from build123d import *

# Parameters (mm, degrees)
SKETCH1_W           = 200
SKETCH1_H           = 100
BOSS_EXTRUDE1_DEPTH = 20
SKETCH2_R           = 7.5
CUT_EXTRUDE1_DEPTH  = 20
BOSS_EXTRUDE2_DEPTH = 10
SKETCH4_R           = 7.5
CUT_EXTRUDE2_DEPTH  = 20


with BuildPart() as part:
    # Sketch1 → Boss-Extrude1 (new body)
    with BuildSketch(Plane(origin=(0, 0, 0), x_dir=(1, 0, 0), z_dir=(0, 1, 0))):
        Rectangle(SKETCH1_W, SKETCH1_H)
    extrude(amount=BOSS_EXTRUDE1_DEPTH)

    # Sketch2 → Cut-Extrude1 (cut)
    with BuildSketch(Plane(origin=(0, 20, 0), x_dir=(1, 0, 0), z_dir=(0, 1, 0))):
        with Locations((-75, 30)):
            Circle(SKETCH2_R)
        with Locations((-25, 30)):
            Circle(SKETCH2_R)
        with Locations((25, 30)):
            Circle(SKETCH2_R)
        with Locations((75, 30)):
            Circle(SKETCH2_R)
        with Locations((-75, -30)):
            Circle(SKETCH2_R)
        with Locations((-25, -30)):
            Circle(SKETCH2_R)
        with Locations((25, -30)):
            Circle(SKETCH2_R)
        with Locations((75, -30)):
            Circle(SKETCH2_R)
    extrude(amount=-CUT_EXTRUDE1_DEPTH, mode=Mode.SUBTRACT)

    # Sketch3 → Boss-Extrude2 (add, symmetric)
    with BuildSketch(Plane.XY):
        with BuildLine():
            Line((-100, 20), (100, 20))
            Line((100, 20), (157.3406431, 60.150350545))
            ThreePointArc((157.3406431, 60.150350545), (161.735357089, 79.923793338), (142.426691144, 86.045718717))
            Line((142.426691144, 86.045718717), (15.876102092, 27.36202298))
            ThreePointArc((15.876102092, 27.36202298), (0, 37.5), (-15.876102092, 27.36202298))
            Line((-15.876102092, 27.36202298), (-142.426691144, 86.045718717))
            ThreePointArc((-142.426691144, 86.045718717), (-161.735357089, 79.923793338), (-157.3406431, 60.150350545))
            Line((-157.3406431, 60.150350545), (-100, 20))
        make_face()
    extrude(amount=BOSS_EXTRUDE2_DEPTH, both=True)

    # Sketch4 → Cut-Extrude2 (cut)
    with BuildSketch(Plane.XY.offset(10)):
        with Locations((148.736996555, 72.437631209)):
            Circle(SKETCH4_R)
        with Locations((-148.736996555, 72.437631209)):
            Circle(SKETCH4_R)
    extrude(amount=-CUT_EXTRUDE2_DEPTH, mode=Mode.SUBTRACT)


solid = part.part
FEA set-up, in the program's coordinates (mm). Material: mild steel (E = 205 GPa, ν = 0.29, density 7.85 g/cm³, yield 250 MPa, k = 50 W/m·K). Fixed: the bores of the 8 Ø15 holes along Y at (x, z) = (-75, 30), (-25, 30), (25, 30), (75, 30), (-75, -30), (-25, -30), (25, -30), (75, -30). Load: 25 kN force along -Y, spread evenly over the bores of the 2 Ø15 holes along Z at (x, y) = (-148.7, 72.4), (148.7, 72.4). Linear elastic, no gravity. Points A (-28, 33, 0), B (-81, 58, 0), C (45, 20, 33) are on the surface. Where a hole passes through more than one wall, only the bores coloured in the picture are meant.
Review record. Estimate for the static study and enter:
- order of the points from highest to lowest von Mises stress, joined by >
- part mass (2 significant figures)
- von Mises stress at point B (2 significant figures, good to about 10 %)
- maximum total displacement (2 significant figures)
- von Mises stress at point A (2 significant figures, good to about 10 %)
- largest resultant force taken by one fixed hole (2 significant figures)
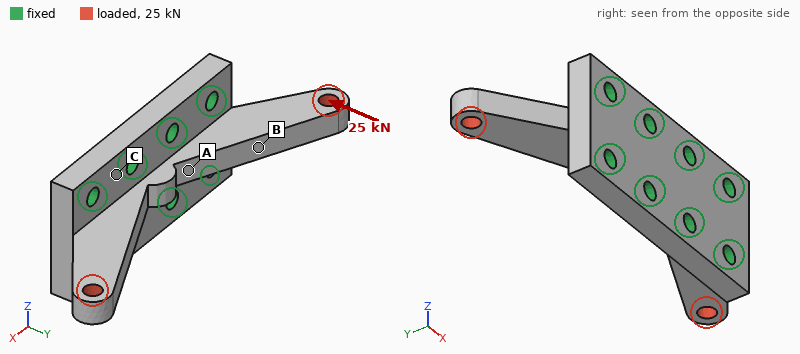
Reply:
B > A > C
4.4 kg
110 MPa
0.18 mm
36 MPa
13 kN
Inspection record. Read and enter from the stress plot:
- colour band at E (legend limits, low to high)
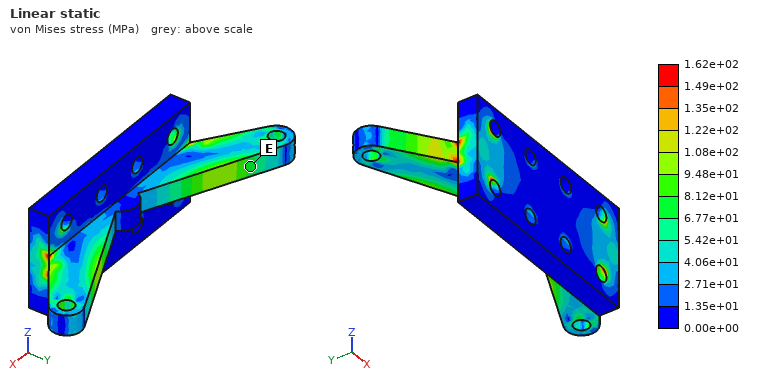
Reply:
6.77e+01 to 8.12e+01 MPa
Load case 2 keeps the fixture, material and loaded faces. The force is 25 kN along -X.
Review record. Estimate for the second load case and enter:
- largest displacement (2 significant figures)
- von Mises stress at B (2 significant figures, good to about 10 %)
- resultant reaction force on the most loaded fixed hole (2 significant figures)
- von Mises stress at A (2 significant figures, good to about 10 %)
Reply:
0.11 mm
80 MPa
6.1 kN
33 MPa
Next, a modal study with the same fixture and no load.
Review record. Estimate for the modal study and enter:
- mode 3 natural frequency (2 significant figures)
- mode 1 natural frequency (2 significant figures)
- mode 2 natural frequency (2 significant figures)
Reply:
3300 Hz
2000 Hz
2000 Hz
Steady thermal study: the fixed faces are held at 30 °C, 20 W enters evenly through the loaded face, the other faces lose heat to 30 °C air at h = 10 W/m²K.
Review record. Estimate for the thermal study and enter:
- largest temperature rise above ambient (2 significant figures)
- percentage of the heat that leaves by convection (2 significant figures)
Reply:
26 K
16 %
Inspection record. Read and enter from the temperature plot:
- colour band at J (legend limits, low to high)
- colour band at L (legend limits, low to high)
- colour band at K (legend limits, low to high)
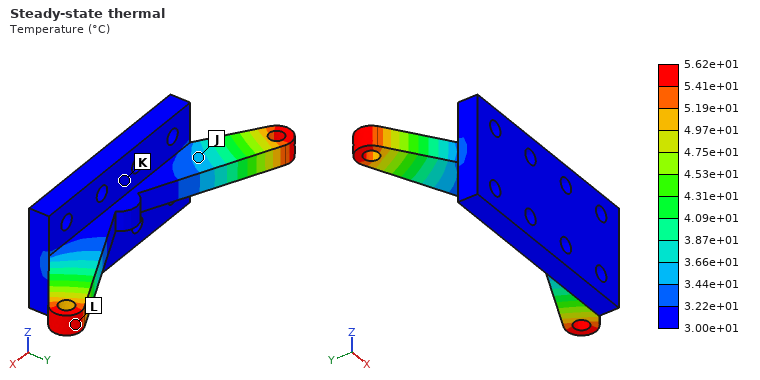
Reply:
3.44e+01 to 3.66e+01 °C
5.41e+01 to 5.62e+01 °C
3.00e+01 to 3.22e+01 °C
